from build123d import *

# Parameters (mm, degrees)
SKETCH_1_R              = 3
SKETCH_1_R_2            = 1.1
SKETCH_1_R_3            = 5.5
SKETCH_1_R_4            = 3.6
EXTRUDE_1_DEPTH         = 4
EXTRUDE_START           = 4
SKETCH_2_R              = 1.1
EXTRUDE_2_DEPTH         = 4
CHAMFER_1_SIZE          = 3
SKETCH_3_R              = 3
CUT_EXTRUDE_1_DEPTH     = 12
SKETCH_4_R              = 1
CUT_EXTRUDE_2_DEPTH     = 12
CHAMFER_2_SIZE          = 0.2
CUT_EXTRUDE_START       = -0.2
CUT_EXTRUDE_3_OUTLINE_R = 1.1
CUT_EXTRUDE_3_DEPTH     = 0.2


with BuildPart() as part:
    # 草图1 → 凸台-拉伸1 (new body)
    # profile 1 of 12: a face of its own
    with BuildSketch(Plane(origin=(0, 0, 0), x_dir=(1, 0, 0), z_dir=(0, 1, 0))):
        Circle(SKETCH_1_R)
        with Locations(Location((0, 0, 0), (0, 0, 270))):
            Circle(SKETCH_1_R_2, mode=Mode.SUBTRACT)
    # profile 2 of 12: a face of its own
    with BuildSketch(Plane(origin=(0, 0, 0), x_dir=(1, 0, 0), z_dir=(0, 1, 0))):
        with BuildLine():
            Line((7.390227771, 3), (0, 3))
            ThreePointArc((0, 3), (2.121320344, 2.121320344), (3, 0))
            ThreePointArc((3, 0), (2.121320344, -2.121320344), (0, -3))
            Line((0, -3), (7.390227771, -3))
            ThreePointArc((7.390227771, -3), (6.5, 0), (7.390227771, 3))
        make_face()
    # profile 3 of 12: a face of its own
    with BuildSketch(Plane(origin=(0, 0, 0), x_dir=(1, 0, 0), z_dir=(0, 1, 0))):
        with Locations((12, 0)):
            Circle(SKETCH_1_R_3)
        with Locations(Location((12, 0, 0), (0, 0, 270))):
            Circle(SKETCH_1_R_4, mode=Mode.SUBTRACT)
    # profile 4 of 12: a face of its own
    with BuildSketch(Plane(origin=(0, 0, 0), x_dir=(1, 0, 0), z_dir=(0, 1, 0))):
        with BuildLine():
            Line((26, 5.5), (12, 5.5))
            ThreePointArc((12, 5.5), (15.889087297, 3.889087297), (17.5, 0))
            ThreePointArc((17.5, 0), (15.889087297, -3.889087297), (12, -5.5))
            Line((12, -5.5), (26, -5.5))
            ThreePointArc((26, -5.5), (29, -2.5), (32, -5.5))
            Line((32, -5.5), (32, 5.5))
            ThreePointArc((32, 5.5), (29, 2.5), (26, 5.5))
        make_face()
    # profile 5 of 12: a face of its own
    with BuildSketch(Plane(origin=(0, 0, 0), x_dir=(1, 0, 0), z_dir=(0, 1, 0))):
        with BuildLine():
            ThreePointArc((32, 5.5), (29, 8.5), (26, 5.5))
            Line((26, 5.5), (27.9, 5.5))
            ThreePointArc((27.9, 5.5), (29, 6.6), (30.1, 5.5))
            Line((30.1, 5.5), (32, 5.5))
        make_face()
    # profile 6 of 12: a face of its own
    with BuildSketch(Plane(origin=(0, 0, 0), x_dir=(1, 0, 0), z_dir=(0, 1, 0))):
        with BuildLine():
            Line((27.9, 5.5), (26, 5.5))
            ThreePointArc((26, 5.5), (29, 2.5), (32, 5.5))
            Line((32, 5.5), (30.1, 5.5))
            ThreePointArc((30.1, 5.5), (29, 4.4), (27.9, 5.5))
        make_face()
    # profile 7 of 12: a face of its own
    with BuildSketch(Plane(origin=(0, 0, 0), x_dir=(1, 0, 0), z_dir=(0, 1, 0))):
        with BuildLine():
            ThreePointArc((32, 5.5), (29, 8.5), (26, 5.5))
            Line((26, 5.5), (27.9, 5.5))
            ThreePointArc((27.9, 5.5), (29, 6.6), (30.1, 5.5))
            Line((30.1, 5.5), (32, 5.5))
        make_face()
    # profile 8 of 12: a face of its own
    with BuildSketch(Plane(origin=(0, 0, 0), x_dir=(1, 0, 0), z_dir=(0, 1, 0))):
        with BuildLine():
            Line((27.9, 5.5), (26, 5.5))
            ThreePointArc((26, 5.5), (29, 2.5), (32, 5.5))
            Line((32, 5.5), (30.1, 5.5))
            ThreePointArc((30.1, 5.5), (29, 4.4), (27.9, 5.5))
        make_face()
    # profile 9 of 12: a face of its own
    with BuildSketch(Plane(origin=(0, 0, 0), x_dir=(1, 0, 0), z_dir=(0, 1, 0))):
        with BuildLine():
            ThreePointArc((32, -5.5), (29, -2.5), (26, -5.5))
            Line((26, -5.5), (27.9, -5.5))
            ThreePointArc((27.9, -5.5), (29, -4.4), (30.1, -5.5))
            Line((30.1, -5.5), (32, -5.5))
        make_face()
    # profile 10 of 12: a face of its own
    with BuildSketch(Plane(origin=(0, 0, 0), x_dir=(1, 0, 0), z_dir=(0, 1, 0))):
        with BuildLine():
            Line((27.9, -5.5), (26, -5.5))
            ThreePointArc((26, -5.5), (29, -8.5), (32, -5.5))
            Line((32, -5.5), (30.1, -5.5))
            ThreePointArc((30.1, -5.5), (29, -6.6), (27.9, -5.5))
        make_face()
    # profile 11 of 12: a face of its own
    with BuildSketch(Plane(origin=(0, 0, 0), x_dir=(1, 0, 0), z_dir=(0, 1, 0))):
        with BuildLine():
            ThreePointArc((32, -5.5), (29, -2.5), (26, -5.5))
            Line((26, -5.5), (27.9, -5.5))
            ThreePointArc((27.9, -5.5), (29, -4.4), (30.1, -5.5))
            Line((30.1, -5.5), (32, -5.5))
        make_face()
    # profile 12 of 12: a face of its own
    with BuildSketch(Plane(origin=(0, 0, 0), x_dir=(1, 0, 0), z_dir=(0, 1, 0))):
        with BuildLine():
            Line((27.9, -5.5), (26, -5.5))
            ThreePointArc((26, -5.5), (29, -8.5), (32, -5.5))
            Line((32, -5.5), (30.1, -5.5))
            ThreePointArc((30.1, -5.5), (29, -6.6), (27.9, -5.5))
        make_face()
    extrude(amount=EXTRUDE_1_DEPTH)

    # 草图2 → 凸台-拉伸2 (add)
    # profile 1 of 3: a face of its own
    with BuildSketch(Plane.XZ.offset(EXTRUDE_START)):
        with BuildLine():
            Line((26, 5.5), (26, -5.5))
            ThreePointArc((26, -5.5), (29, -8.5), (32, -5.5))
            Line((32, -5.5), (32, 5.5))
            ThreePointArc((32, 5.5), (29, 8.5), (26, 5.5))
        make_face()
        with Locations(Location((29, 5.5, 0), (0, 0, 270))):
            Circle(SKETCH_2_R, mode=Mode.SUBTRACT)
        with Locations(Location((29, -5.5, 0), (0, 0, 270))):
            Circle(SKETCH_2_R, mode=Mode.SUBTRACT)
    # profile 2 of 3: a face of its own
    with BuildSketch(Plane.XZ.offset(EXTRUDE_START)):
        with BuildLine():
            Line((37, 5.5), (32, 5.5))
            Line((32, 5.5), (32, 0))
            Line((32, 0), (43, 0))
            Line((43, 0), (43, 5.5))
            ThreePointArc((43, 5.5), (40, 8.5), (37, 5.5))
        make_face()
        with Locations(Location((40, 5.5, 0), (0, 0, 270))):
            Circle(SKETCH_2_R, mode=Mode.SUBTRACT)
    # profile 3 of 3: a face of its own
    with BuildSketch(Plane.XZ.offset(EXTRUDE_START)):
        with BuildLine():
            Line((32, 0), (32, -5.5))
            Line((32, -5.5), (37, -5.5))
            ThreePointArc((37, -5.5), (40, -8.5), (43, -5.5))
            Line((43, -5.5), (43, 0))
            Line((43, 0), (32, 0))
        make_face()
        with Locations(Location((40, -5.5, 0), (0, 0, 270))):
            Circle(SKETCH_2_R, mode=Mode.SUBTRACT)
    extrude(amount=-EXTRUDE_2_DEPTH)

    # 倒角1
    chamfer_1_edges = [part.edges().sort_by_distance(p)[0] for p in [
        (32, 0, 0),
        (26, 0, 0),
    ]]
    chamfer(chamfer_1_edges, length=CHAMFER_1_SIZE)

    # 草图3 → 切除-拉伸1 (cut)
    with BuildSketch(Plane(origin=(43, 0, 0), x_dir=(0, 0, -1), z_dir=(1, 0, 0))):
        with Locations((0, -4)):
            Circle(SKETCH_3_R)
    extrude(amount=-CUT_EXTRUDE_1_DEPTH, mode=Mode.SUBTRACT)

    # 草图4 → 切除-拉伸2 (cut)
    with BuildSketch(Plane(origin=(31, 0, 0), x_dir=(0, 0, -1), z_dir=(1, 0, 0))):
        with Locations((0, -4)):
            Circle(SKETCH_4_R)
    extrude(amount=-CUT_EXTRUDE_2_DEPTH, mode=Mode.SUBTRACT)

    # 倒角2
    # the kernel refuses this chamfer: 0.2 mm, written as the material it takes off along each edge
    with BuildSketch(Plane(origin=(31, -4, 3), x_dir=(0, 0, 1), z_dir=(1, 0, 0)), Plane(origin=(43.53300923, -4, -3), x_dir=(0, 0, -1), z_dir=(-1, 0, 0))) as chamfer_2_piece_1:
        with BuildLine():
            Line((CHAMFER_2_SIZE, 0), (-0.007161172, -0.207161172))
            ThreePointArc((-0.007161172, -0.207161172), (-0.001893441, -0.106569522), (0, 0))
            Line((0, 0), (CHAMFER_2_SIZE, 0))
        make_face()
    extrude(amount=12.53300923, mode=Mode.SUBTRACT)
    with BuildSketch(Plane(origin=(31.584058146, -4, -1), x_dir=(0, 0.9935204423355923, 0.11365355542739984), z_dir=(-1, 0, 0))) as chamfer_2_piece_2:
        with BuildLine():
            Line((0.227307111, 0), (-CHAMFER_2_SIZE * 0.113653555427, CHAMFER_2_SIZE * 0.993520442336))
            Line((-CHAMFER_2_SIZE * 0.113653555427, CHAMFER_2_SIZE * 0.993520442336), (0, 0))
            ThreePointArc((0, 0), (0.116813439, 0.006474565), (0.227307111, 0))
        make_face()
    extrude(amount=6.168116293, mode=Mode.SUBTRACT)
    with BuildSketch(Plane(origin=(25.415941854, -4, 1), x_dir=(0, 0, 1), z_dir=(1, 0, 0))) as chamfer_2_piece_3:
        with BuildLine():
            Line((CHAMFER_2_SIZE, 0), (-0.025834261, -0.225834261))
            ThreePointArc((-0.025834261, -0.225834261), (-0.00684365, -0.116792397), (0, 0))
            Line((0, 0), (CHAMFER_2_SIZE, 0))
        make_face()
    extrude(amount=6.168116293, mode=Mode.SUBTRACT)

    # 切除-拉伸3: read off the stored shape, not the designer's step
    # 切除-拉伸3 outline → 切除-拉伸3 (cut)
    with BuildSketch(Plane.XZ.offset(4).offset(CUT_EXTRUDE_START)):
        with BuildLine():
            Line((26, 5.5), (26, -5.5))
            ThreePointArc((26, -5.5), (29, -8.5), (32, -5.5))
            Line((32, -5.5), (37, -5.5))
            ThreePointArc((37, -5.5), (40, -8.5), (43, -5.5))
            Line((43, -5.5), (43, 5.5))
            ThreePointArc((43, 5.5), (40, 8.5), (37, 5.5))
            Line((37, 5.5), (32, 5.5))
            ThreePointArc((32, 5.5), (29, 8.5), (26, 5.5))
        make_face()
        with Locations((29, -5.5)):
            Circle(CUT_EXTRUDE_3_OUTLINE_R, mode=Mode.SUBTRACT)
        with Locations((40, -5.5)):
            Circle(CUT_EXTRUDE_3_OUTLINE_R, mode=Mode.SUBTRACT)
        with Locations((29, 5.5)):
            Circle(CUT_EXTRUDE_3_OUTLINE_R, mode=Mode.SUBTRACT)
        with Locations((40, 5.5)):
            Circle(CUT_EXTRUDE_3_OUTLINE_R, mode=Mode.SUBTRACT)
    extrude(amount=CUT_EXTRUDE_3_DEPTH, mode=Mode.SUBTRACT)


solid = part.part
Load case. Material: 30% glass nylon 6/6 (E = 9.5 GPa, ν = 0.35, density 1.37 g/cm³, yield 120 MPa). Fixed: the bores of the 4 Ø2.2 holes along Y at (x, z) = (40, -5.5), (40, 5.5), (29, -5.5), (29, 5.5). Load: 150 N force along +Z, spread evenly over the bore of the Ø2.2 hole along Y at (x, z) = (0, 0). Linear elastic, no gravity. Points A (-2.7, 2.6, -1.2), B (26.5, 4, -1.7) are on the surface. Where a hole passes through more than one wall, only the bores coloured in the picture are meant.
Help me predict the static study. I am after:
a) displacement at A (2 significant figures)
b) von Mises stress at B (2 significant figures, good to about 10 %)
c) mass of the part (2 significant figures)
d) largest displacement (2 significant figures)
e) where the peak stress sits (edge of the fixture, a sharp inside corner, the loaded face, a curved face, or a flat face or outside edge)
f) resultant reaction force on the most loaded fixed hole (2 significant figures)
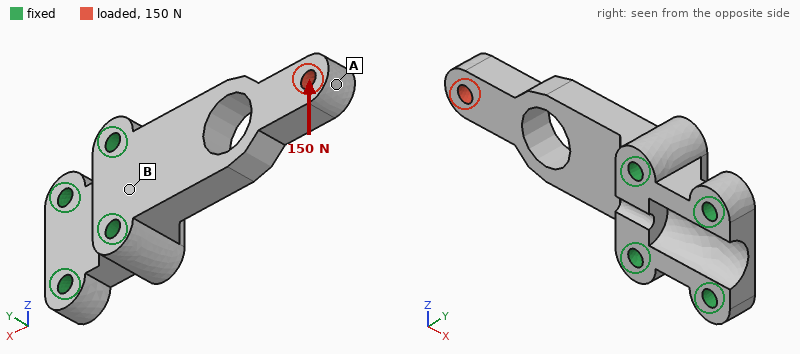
0.45 mm
10 MPa
2.7 g
0.46 mm
a curved face
400 N
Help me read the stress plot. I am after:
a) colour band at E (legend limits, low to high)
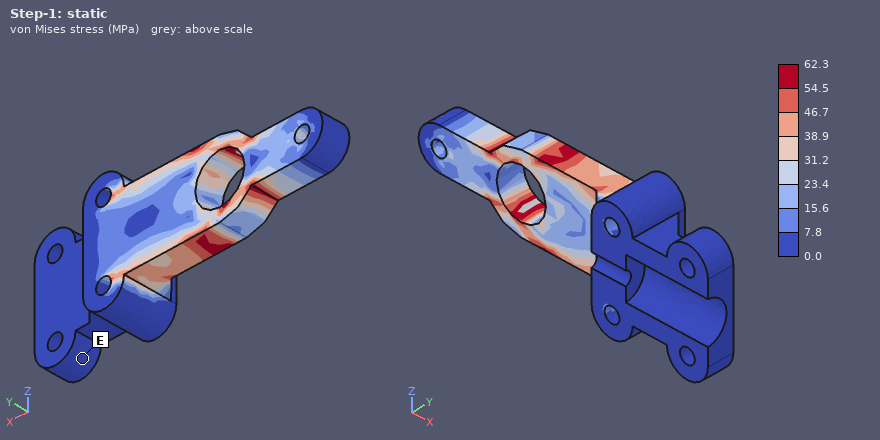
0.0 to 7.8 MPa
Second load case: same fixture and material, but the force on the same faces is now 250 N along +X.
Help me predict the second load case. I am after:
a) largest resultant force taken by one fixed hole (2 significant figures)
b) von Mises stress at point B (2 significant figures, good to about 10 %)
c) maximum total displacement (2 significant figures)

120 N
4.2 MPa
59 µm
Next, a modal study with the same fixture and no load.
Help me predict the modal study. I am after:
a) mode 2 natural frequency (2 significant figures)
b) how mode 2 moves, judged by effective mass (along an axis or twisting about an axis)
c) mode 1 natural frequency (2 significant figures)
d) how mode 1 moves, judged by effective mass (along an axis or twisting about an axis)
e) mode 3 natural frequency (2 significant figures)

5900 Hz
along Z
2600 Hz
along Y
11 kHz
